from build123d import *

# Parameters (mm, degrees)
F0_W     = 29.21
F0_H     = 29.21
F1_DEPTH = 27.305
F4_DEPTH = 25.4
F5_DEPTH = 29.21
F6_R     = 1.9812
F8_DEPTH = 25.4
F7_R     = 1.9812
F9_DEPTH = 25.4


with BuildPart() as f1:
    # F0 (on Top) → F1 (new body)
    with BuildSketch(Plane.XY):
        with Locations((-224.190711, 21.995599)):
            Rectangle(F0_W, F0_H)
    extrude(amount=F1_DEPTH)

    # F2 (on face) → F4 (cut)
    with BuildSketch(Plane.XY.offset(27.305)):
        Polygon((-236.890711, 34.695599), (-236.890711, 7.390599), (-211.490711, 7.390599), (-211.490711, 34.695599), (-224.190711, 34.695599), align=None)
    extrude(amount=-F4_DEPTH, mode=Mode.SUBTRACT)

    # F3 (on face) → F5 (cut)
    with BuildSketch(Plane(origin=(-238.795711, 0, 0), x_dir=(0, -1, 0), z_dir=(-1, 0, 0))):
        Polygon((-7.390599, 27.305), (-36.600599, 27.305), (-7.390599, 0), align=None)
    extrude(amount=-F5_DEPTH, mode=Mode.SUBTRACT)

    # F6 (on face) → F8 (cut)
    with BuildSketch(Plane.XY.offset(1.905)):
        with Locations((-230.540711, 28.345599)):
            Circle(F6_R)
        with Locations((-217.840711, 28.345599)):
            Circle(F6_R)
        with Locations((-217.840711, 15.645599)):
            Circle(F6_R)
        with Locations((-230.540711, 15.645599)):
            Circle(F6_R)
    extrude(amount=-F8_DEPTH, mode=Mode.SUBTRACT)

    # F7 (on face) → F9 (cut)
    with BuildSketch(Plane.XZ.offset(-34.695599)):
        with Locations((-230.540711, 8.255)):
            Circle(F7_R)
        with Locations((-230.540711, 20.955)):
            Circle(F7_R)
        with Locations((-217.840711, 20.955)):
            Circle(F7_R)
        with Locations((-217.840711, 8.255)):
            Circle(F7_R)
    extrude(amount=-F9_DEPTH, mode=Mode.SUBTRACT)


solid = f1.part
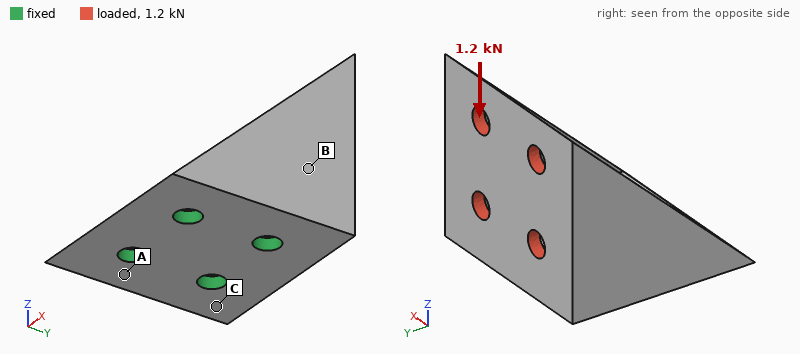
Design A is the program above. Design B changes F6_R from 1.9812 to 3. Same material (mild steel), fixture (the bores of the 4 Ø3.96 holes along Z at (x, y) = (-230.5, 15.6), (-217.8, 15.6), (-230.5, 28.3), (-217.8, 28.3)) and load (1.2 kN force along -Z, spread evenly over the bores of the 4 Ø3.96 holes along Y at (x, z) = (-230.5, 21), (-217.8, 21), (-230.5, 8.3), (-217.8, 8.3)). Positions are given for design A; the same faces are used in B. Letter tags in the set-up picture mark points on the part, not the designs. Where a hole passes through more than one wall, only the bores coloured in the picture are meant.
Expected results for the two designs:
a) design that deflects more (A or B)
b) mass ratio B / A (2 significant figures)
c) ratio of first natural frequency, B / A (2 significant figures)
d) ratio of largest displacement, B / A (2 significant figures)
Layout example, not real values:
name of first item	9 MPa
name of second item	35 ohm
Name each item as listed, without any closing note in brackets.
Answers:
design that deflects more	A
mass ratio B / A	0.97
ratio of first natural frequency, B / A	1.3
ratio of largest displacement, B / A	0.62
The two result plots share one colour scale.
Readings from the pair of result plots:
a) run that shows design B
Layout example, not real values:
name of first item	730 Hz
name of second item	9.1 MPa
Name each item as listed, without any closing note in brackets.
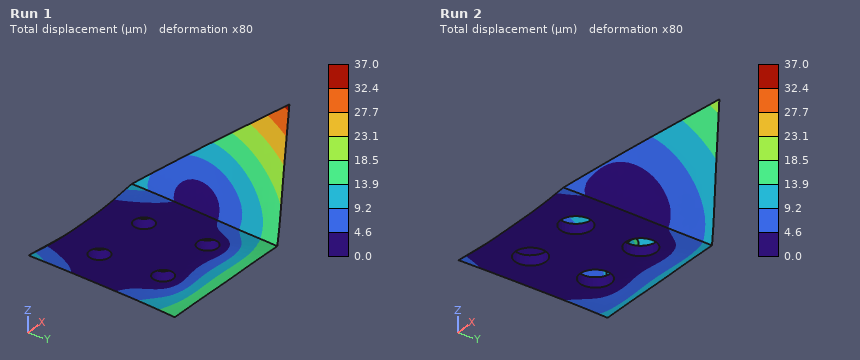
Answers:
run that shows design B	Run 2
